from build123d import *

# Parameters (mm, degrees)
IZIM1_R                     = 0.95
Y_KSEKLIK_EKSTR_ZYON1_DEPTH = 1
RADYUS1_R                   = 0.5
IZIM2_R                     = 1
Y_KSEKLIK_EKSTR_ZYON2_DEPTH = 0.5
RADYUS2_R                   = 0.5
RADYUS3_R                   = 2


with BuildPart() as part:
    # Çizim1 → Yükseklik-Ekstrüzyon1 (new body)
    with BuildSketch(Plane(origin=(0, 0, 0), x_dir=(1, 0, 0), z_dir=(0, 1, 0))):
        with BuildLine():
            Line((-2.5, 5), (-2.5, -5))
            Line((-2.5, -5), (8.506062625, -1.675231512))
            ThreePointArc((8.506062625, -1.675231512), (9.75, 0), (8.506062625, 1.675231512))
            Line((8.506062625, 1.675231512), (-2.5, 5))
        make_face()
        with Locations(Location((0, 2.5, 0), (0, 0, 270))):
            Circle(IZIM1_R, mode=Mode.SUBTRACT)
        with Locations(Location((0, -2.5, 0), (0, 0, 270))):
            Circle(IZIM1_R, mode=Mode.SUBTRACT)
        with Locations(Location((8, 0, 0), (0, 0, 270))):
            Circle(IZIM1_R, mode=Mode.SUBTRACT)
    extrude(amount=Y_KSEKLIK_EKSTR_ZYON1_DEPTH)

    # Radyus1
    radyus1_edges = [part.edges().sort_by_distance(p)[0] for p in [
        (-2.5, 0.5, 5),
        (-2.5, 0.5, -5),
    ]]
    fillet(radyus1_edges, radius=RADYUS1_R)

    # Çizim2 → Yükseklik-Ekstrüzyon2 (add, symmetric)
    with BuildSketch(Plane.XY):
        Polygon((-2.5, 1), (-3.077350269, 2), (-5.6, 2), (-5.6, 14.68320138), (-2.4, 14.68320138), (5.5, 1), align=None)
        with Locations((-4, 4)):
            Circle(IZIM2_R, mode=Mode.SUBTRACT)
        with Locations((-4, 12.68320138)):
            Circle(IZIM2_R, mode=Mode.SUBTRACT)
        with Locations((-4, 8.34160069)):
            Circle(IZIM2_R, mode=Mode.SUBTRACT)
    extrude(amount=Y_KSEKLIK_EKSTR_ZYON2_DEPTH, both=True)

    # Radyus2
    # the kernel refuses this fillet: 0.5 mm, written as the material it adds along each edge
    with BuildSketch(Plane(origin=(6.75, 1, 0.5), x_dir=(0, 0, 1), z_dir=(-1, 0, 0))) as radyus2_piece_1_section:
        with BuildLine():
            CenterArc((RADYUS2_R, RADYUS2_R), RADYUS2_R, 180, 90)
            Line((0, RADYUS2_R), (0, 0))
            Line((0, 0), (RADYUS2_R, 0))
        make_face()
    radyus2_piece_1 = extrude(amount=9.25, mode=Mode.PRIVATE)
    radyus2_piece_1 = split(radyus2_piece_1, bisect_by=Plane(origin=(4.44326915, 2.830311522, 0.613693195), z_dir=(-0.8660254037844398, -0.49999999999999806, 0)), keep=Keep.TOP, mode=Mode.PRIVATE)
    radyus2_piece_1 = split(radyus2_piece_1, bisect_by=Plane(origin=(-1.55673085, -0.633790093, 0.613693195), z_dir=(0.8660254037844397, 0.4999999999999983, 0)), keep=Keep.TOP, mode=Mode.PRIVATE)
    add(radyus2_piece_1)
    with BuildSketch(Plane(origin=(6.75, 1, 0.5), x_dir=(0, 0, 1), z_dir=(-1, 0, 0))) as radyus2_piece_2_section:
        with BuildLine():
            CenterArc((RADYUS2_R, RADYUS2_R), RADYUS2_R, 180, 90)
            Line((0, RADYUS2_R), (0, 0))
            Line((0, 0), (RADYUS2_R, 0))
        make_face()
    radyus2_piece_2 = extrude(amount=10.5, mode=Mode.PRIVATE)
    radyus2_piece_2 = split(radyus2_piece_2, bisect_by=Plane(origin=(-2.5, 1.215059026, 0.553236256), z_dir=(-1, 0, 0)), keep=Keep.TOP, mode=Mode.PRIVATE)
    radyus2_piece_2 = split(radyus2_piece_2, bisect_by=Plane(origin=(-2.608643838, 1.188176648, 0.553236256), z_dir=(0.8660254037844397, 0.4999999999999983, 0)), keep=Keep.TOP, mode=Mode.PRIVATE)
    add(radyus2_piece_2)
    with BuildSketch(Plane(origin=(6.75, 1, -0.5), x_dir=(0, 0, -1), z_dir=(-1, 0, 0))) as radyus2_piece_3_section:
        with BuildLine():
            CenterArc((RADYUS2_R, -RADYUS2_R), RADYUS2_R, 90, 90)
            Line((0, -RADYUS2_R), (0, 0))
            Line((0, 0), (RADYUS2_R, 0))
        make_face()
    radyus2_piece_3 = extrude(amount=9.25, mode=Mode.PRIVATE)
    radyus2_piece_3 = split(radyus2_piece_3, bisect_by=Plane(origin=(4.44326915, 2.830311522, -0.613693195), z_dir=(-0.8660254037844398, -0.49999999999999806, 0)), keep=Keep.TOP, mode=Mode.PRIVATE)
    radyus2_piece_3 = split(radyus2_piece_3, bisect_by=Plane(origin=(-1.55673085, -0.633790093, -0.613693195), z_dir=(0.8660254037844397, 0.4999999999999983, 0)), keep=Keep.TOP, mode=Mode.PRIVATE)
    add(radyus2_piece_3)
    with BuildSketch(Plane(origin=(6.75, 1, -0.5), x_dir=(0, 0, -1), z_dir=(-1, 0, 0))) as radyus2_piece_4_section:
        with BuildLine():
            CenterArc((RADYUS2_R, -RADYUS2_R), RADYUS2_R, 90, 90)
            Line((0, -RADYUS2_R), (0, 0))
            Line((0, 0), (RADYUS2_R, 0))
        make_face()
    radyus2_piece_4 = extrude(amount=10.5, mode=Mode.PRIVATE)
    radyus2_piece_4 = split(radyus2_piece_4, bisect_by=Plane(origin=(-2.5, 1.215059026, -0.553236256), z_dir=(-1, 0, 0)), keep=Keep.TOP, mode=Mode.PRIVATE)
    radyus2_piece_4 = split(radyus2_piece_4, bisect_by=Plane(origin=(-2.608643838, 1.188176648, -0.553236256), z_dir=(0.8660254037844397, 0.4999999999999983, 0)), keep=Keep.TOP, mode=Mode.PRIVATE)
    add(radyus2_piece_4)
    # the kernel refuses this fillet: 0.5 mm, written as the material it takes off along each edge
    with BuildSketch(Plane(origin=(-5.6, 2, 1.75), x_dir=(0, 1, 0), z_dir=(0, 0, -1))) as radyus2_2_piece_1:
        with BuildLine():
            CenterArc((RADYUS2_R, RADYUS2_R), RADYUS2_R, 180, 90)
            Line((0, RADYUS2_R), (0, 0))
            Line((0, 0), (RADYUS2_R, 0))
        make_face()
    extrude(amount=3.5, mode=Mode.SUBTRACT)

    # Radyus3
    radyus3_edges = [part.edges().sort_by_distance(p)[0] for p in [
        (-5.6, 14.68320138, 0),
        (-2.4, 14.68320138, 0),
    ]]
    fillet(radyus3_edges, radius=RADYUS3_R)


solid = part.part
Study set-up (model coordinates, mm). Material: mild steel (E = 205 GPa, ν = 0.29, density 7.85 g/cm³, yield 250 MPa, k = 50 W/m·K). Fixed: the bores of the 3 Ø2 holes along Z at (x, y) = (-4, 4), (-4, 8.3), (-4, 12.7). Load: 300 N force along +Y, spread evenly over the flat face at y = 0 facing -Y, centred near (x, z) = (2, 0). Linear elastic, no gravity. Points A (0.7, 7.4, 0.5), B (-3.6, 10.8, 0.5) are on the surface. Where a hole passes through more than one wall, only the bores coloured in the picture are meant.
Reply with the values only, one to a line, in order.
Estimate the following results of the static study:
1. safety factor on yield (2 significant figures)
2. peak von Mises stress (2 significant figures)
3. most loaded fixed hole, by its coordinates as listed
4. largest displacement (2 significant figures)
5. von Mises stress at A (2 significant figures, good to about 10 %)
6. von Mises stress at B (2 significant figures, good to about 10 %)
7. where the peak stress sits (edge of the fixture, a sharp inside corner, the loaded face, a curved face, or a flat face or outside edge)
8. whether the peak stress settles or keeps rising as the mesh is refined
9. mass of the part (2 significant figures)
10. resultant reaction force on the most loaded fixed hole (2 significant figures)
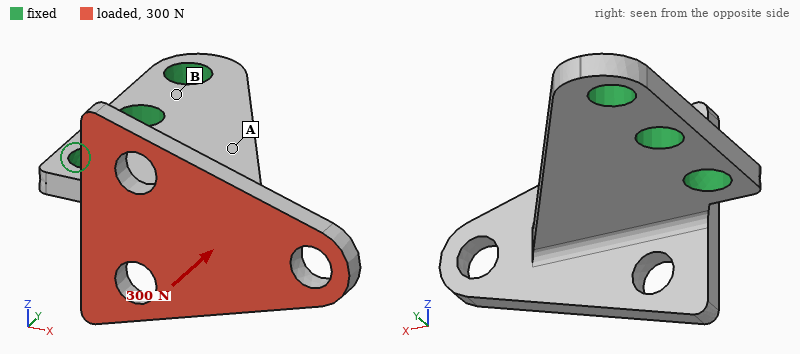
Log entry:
0.90
280 MPa
(-4, 4)
28 µm
92 MPa
27 MPa
a curved face
settles
1.2 g
250 N
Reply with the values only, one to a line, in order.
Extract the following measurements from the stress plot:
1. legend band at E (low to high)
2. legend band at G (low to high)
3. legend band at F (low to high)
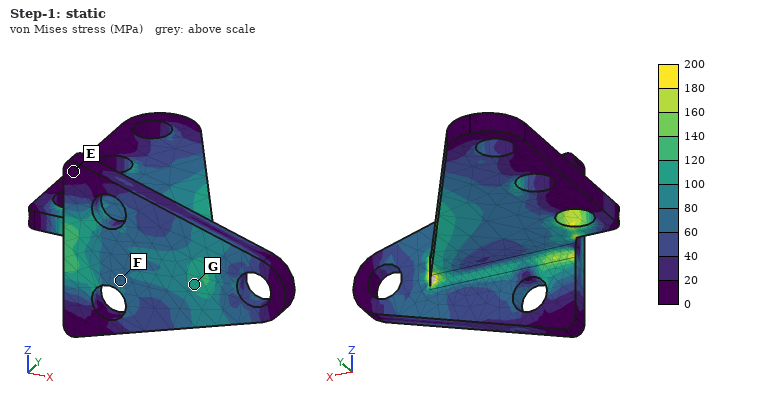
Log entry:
0 to 20 MPa
100 to 120 MPa
60 to 80 MPa
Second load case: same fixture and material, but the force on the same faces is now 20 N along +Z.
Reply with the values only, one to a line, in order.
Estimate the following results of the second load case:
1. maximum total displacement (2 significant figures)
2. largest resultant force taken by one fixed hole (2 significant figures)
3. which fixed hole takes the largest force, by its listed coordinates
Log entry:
40 µm
28 N
(-4, 4)
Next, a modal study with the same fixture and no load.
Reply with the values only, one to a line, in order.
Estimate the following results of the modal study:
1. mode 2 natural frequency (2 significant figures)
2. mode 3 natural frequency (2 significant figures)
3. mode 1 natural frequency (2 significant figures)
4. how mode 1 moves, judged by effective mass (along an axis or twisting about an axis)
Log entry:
17 kHz
29 kHz
5900 Hz
along Z
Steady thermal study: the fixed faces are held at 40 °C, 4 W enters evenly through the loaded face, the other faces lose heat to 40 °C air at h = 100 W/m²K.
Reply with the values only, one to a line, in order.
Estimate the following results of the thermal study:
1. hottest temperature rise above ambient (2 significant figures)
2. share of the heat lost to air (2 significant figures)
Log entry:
68 K
23 %
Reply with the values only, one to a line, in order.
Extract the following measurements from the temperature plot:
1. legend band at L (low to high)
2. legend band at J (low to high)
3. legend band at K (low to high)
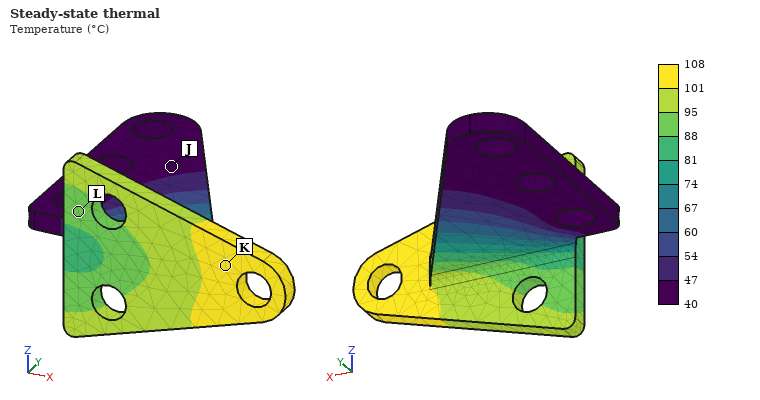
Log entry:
88 to 95 °C
40 to 47 °C
101 to 108 °C
